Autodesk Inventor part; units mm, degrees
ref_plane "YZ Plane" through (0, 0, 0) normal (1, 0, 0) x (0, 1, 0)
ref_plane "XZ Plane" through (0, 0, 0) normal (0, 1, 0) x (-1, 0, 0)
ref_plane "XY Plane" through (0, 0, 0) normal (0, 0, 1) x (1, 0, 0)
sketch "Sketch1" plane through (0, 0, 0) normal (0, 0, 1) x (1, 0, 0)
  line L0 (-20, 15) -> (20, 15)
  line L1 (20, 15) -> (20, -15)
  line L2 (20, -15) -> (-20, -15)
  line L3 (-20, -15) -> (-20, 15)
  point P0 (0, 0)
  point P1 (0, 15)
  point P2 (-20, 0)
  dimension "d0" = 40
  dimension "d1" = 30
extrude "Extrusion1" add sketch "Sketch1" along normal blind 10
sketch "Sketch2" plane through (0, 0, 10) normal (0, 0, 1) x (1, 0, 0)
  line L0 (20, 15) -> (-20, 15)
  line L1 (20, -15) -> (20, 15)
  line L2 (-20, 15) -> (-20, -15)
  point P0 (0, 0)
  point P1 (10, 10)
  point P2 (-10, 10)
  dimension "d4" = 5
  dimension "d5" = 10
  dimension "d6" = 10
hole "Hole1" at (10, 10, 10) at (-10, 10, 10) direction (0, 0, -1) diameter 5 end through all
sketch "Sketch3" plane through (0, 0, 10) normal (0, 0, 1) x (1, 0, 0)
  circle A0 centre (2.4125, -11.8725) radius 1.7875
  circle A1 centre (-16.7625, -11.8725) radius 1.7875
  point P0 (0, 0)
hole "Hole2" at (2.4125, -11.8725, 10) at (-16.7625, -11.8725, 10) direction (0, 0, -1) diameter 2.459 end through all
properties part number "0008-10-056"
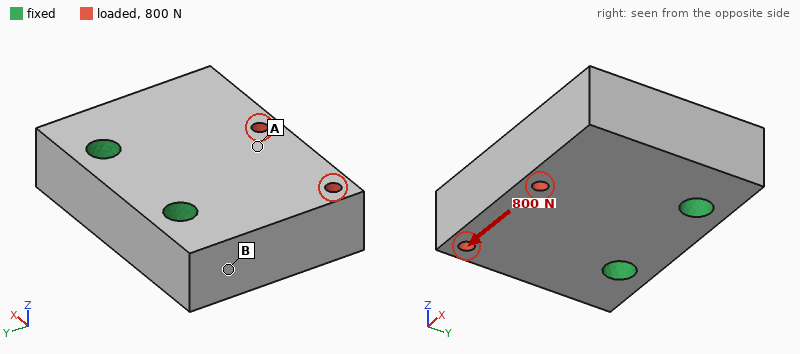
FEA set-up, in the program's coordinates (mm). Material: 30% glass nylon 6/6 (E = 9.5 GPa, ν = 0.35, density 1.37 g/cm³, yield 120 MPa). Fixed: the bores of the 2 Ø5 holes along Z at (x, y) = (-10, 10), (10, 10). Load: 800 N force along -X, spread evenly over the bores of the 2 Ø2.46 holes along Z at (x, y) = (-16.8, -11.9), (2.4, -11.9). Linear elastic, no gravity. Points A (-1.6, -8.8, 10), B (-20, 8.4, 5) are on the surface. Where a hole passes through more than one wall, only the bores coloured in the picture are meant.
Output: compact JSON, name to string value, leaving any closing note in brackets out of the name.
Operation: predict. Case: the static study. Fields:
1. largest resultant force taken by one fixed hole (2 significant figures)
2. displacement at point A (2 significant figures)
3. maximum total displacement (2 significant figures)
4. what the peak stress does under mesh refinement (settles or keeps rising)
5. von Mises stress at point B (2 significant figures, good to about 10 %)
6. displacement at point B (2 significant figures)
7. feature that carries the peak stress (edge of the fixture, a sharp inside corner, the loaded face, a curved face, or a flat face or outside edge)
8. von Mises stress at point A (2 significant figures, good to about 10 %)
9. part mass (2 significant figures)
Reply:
{"largest resultant force taken by one fixed hole": "810 N", "displacement at point A": "22 µm", "maximum total displacement": "39 µm", "what the peak stress does under mesh refinement": "keeps rising", "von Mises stress at point B": "2.5 MPa", "displacement at point B": "12 µm", "feature that carries the peak stress": "edge of the fixture", "von Mises stress at point A": "5.7 MPa", "part mass": "16 g"}
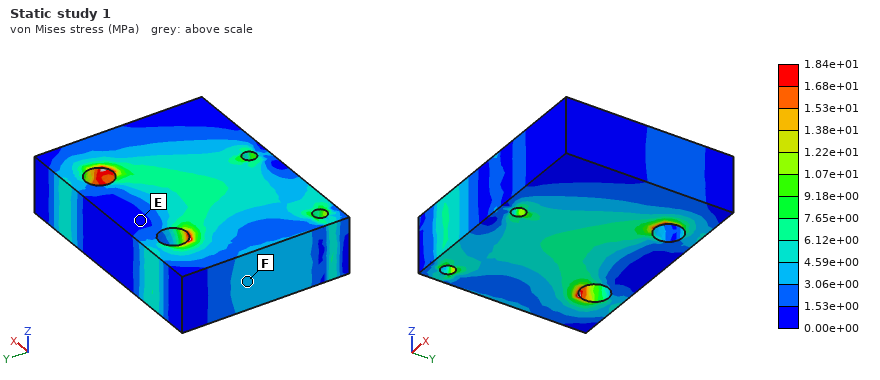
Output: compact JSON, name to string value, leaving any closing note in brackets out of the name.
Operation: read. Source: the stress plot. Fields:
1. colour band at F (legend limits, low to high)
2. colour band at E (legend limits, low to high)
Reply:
{"colour band at F": "3.06e+00 to 4.59e+00 MPa", "colour band at E": "0.00e+00 to 1.53e+00 MPa"}
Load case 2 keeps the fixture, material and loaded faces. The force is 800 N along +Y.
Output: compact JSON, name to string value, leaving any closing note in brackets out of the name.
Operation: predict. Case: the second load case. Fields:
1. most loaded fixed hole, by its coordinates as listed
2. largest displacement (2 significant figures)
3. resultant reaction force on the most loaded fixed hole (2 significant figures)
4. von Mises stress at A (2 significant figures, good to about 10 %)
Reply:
{"most loaded fixed hole, by its coordinates as listed": "(-10, 10)", "largest displacement": "17 µm", "resultant reaction force on the most loaded fixed hole": "640 N", "von Mises stress at A": "3.7 MPa"}
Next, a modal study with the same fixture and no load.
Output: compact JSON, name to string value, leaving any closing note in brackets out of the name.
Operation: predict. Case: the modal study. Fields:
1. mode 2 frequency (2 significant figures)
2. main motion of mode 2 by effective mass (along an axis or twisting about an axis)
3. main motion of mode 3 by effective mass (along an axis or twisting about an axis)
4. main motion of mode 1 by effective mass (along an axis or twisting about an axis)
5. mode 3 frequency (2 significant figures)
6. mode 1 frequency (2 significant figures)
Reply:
{"mode 2 frequency": "9100 Hz", "main motion of mode 2 by effective mass": "twisting about Y", "main motion of mode 3 by effective mass": "along X", "main motion of mode 1 by effective mass": "along Z", "mode 3 frequency": "11 kHz", "mode 1 frequency": "6000 Hz"}
